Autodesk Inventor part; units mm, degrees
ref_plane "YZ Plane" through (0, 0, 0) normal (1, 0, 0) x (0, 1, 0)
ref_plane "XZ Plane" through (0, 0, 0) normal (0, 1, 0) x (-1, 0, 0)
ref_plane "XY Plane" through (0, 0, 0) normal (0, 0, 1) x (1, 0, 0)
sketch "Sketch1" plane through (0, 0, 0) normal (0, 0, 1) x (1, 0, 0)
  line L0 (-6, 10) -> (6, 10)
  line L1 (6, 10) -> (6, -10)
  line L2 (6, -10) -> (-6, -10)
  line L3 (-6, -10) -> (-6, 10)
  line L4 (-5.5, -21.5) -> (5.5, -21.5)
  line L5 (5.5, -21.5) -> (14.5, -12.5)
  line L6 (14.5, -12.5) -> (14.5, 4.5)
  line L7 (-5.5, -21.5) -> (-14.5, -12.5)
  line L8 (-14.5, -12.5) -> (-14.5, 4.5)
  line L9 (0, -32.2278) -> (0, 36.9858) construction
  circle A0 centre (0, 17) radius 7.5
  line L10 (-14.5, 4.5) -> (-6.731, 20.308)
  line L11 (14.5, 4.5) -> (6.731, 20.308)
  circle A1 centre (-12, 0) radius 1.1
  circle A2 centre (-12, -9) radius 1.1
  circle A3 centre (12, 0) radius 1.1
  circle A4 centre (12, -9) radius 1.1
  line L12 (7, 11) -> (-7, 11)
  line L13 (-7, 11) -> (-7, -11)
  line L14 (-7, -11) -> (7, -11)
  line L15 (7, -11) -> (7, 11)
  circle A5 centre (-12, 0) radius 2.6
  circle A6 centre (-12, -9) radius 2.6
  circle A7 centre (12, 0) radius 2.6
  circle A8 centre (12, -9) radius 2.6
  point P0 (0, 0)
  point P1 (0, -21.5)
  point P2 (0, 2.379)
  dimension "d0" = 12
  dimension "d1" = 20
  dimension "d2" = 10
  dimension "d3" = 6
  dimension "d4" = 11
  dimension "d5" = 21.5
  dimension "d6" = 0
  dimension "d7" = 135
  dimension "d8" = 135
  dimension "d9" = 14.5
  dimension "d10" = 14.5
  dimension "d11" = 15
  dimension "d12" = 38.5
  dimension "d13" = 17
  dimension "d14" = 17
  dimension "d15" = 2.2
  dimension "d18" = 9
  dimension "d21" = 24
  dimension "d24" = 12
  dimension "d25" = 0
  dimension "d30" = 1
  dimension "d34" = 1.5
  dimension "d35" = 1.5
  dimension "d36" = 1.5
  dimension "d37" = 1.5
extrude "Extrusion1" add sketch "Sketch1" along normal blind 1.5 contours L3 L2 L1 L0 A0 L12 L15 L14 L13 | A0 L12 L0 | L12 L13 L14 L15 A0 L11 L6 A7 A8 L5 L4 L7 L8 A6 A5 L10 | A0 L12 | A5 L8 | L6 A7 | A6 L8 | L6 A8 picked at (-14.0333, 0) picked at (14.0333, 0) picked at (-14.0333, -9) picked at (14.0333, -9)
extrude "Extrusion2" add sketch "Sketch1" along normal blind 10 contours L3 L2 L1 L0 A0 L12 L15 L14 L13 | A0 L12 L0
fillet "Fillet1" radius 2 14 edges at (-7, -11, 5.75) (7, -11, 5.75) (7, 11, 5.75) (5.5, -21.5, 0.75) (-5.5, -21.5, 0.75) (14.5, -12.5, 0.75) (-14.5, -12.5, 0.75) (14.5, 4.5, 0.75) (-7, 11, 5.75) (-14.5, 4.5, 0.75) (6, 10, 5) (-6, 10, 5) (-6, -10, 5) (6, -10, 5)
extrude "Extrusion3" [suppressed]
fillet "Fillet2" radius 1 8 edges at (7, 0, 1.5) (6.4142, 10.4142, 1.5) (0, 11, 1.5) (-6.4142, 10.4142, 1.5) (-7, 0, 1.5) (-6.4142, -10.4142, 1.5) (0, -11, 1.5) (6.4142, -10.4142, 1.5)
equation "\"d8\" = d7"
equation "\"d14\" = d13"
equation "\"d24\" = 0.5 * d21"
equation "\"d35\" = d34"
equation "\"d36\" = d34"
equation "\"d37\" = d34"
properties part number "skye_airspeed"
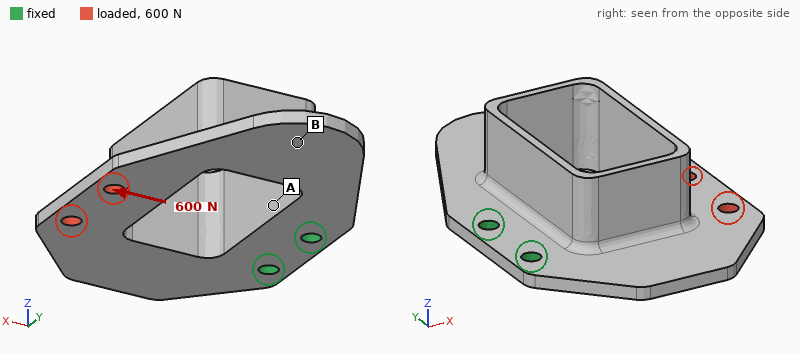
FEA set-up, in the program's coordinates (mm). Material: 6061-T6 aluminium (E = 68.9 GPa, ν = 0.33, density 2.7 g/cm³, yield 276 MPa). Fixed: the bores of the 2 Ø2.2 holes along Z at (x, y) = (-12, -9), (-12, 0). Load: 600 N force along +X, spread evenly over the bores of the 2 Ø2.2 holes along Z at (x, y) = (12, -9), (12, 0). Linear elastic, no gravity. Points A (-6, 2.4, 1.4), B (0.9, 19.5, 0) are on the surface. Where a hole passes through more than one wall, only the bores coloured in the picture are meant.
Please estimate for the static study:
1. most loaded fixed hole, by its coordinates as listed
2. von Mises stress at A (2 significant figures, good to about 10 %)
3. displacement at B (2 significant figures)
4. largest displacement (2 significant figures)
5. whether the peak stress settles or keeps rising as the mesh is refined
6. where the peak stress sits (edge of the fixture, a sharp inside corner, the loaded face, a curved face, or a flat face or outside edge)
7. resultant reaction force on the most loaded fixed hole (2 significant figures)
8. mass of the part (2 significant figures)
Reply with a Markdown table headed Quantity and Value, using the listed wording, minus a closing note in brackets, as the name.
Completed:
| Quantity | Value |
|---|---|
| most loaded fixed hole, by its coordinates as listed | (-12, -9) |
| von Mises stress at A | 48 MPa |
| displacement at B | 39 µm |
| largest displacement | 70 µm |
| whether the peak stress settles or keeps rising as the mesh is refined | keeps rising |
| where the peak stress sits | edge of the fixture |
| resultant reaction force on the most loaded fixed hole | 360 N |
| mass of the part | 4.8 g |
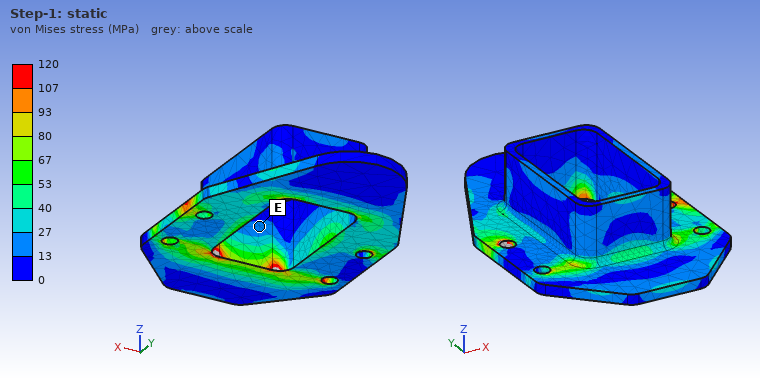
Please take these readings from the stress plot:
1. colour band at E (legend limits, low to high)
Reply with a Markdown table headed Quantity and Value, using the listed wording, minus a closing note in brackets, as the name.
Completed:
| Quantity | Value |
|---|---|
| colour band at E | 13 to 27 MPa |
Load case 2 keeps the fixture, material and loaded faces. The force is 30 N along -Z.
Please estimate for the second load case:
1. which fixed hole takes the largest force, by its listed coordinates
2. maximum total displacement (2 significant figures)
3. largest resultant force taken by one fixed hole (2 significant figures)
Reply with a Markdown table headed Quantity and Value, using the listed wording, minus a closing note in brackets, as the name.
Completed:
| Quantity | Value |
|---|---|
| which fixed hole takes the largest force, by its listed coordinates | (-12, 0) |
| maximum total displacement | 0.26 mm |
| largest resultant force taken by one fixed hole | 27 N |
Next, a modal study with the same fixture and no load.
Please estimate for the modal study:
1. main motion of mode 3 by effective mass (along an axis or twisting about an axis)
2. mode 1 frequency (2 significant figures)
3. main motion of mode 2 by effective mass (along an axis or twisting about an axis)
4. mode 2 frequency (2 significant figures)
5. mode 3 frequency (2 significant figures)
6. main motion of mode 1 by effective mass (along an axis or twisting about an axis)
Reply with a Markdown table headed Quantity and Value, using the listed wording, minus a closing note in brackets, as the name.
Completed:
| Quantity | Value |
|---|---|
| main motion of mode 3 by effective mass | along Y |
| mode 1 frequency | 1500 Hz |
| main motion of mode 2 by effective mass | twisting about X |
| mode 2 frequency | 2600 Hz |
| mode 3 frequency | 5400 Hz |
| main motion of mode 1 by effective mass | along Z |
